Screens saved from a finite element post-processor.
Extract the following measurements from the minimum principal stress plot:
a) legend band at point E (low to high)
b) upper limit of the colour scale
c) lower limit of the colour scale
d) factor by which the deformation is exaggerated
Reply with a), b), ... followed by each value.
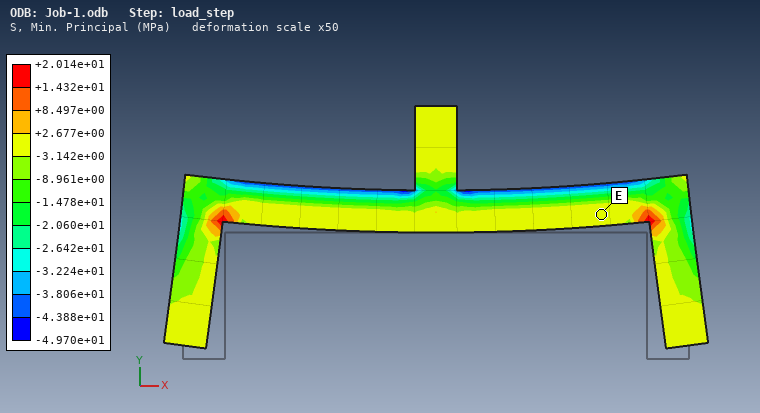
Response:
a) -3.142e+00 to +2.677e+00 MPa
b) +2.014e+01 MPa
c) -4.970e+01 MPa
d) 50
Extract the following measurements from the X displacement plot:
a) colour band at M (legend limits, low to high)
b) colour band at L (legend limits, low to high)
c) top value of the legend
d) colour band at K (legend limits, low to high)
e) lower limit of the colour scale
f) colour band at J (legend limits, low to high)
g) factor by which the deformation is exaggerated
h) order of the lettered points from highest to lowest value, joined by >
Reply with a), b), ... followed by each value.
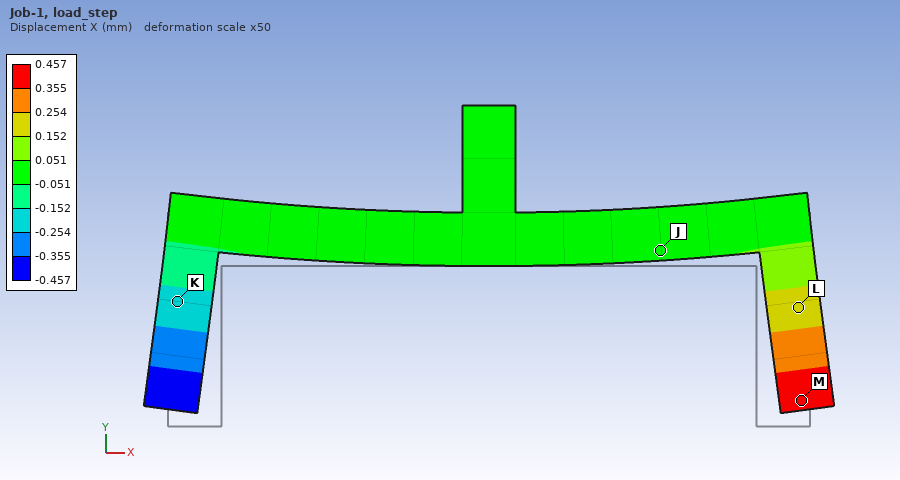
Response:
a) 0.355 to 0.457 mm
b) 0.152 to 0.254 mm
c) 0.457 mm
d) -0.254 to -0.152 mm
e) -0.457 mm
f) -0.051 to 0.051 mm
g) 50
h) M > L > J > K
